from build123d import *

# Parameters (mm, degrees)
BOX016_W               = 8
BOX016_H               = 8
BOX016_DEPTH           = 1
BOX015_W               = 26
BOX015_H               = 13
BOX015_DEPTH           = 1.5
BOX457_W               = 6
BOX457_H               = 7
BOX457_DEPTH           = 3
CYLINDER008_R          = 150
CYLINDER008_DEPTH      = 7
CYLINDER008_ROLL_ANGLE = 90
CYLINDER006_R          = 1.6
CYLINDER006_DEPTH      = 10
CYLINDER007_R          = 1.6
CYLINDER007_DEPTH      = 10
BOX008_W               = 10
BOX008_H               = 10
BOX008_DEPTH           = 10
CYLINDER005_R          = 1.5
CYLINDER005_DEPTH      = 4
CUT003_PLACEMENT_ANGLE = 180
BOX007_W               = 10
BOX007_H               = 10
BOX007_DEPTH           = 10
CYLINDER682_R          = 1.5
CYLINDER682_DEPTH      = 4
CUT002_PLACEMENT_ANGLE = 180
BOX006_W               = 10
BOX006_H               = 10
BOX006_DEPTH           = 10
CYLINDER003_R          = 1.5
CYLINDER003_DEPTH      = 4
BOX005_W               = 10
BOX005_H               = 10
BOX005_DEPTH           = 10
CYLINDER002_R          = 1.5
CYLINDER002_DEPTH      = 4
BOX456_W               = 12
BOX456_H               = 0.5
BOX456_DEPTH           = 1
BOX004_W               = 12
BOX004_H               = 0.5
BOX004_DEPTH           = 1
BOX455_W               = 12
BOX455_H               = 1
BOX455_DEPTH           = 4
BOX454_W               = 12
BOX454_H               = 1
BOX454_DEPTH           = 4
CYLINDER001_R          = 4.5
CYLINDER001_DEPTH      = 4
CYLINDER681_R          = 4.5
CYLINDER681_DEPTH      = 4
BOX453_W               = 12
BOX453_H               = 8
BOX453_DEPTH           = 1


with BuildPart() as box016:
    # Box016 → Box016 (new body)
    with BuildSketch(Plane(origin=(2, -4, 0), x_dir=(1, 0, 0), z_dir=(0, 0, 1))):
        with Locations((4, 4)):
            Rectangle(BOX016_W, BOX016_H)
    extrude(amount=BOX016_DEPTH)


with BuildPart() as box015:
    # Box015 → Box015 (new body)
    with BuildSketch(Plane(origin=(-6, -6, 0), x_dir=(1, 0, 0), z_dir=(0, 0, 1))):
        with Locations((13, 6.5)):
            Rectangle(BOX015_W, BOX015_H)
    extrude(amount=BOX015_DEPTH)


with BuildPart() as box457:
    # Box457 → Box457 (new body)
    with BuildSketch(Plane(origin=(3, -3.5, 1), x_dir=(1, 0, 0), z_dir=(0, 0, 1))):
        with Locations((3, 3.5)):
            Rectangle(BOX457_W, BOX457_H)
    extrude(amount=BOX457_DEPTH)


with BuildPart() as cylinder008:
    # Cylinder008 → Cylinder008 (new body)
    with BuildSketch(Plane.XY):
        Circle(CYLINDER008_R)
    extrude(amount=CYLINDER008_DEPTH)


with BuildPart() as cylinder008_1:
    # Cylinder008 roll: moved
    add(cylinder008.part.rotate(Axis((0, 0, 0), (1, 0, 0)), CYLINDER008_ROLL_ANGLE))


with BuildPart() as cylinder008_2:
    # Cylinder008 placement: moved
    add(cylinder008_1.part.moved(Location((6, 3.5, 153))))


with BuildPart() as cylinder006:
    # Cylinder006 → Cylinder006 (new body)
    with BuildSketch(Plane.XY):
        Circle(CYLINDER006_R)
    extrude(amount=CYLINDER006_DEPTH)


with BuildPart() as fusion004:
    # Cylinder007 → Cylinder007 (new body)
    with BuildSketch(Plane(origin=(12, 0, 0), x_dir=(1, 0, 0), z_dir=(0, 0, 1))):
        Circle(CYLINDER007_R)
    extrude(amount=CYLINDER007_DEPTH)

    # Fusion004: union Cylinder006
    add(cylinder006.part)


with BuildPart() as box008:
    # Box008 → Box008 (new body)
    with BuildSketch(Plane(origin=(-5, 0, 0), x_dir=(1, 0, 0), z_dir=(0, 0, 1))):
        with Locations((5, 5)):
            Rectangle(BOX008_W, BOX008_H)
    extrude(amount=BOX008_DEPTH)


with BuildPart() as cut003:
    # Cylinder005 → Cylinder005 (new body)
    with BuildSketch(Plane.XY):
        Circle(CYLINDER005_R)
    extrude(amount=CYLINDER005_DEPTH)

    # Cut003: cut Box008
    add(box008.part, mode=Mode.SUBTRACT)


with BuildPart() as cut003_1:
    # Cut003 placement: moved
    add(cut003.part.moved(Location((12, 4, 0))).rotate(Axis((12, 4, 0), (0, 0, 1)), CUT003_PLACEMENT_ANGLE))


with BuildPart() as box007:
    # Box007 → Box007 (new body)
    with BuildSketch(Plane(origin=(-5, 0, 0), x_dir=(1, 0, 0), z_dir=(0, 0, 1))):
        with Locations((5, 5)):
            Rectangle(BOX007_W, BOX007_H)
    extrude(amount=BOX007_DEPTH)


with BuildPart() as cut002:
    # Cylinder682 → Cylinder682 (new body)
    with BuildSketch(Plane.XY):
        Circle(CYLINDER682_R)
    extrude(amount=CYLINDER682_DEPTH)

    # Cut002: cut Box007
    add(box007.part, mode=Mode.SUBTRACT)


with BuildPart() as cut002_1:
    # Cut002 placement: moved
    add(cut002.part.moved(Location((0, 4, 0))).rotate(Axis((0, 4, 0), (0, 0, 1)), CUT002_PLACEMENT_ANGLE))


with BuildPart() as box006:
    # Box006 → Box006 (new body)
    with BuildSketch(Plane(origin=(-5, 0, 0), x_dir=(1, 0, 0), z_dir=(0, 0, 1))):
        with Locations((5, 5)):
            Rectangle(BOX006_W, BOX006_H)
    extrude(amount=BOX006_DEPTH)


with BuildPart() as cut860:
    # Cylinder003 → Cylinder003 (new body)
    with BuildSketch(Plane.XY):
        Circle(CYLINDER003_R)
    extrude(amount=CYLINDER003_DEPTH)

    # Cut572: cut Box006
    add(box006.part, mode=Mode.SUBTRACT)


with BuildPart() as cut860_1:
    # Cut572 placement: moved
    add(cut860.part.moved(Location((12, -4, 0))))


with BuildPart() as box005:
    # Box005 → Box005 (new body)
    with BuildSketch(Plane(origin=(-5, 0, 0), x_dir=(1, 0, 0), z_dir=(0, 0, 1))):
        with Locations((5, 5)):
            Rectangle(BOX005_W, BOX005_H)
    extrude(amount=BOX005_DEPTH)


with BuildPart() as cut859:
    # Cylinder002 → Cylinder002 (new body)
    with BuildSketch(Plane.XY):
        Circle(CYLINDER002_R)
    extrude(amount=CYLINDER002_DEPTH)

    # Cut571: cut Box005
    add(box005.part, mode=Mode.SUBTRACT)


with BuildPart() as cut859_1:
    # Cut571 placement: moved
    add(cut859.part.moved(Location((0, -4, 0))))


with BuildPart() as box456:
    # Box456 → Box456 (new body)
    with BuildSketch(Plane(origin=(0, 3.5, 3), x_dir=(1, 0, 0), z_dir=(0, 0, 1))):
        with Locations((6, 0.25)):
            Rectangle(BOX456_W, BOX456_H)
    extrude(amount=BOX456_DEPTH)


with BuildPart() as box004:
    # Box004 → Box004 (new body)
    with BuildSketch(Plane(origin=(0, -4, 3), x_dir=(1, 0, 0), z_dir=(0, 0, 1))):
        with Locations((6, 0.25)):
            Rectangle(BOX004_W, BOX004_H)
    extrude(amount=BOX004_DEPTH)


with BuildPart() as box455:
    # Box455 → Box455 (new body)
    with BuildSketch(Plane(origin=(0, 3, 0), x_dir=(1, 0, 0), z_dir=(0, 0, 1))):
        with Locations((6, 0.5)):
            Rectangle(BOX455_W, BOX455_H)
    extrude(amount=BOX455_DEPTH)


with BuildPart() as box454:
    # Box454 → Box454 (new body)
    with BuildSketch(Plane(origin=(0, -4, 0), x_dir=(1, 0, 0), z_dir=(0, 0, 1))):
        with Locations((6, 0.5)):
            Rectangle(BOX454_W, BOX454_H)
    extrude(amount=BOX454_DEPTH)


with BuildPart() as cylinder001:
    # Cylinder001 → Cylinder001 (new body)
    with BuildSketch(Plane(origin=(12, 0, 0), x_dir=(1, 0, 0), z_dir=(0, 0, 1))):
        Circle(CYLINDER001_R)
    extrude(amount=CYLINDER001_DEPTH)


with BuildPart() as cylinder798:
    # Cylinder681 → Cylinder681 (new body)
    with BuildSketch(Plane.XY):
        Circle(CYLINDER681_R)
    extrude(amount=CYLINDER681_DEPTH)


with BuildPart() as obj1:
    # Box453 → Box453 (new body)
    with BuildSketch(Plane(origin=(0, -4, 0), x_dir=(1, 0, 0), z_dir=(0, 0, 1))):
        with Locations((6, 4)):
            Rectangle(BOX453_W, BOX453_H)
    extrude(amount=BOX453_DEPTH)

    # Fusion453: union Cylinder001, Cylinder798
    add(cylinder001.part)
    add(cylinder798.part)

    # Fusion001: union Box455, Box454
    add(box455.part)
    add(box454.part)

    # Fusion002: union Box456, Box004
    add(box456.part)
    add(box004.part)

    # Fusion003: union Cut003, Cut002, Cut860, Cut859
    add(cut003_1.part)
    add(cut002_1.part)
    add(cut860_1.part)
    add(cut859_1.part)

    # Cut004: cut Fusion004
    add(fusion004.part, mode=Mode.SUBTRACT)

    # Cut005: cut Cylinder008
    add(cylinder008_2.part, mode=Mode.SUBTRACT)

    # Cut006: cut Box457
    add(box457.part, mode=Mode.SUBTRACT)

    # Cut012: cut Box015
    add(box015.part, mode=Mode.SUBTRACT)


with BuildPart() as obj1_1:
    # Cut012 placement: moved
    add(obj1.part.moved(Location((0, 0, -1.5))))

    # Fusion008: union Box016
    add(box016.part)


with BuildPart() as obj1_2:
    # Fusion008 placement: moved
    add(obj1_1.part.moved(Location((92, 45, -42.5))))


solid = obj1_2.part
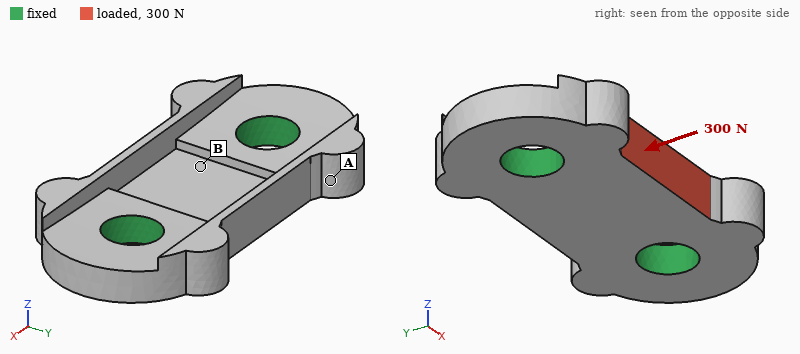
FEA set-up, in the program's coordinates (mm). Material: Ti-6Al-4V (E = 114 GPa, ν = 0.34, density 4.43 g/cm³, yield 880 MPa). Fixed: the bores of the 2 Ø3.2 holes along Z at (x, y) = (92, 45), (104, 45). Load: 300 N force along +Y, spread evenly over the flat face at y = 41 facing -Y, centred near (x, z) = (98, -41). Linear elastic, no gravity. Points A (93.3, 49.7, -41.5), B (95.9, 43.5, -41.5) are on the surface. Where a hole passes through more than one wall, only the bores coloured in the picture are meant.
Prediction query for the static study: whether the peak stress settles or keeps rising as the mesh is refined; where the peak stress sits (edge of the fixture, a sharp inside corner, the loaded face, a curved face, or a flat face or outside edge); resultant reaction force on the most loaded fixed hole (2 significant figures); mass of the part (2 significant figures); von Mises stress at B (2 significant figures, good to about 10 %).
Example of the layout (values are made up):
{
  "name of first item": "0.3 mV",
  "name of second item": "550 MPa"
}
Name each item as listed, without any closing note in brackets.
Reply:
{
  "whether the peak stress settles or keeps rising as the mesh is refined": "keeps rising",
  "where the peak stress sits": "a sharp inside corner",
  "resultant reaction force on the most loaded fixed hole": "150 N",
  "mass of the part": "1.1 g",
  "von Mises stress at B": "61 MPa"
}
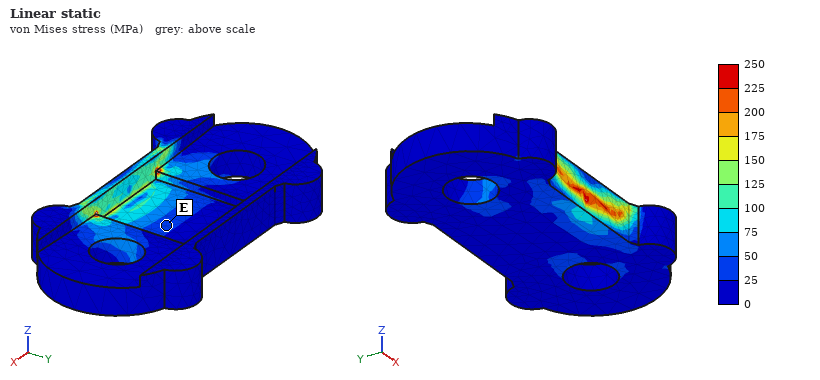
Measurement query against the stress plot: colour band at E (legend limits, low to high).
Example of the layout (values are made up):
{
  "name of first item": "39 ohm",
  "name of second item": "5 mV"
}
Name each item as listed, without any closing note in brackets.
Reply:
{
  "colour band at E": "25 to 50 MPa"
}
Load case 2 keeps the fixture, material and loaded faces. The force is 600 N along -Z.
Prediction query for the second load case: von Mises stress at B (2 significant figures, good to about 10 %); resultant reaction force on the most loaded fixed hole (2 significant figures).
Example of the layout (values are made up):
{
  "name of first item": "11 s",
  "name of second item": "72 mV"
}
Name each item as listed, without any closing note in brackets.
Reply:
{
  "von Mises stress at B": "190 MPa",
  "resultant reaction force on the most loaded fixed hole": "300 N"
}
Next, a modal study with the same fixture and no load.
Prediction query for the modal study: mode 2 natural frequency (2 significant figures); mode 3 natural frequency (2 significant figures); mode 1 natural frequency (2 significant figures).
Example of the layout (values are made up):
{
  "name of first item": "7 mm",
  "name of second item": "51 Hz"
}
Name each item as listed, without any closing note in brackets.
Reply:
{
  "mode 2 natural frequency": "65 kHz",
  "mode 3 natural frequency": "75 kHz",
  "mode 1 natural frequency": "63 kHz"
}
